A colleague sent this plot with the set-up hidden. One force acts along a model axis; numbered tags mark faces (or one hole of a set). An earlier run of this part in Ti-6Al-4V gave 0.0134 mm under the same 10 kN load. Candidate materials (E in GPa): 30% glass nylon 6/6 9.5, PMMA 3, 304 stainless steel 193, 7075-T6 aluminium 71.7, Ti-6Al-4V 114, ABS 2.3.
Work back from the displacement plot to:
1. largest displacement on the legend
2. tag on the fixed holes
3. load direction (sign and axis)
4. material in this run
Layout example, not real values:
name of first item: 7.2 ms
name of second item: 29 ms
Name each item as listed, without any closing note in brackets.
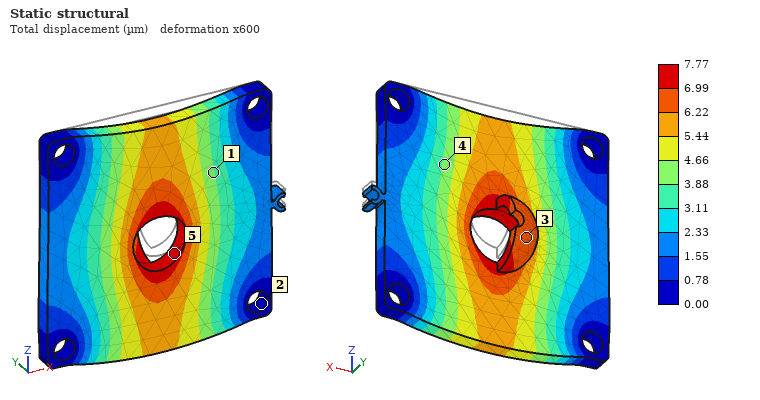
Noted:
largest displacement on the legend: 7.77 µm
tag on the fixed holes: 2
load direction: -Z
material in this run: 304 stainless steel
